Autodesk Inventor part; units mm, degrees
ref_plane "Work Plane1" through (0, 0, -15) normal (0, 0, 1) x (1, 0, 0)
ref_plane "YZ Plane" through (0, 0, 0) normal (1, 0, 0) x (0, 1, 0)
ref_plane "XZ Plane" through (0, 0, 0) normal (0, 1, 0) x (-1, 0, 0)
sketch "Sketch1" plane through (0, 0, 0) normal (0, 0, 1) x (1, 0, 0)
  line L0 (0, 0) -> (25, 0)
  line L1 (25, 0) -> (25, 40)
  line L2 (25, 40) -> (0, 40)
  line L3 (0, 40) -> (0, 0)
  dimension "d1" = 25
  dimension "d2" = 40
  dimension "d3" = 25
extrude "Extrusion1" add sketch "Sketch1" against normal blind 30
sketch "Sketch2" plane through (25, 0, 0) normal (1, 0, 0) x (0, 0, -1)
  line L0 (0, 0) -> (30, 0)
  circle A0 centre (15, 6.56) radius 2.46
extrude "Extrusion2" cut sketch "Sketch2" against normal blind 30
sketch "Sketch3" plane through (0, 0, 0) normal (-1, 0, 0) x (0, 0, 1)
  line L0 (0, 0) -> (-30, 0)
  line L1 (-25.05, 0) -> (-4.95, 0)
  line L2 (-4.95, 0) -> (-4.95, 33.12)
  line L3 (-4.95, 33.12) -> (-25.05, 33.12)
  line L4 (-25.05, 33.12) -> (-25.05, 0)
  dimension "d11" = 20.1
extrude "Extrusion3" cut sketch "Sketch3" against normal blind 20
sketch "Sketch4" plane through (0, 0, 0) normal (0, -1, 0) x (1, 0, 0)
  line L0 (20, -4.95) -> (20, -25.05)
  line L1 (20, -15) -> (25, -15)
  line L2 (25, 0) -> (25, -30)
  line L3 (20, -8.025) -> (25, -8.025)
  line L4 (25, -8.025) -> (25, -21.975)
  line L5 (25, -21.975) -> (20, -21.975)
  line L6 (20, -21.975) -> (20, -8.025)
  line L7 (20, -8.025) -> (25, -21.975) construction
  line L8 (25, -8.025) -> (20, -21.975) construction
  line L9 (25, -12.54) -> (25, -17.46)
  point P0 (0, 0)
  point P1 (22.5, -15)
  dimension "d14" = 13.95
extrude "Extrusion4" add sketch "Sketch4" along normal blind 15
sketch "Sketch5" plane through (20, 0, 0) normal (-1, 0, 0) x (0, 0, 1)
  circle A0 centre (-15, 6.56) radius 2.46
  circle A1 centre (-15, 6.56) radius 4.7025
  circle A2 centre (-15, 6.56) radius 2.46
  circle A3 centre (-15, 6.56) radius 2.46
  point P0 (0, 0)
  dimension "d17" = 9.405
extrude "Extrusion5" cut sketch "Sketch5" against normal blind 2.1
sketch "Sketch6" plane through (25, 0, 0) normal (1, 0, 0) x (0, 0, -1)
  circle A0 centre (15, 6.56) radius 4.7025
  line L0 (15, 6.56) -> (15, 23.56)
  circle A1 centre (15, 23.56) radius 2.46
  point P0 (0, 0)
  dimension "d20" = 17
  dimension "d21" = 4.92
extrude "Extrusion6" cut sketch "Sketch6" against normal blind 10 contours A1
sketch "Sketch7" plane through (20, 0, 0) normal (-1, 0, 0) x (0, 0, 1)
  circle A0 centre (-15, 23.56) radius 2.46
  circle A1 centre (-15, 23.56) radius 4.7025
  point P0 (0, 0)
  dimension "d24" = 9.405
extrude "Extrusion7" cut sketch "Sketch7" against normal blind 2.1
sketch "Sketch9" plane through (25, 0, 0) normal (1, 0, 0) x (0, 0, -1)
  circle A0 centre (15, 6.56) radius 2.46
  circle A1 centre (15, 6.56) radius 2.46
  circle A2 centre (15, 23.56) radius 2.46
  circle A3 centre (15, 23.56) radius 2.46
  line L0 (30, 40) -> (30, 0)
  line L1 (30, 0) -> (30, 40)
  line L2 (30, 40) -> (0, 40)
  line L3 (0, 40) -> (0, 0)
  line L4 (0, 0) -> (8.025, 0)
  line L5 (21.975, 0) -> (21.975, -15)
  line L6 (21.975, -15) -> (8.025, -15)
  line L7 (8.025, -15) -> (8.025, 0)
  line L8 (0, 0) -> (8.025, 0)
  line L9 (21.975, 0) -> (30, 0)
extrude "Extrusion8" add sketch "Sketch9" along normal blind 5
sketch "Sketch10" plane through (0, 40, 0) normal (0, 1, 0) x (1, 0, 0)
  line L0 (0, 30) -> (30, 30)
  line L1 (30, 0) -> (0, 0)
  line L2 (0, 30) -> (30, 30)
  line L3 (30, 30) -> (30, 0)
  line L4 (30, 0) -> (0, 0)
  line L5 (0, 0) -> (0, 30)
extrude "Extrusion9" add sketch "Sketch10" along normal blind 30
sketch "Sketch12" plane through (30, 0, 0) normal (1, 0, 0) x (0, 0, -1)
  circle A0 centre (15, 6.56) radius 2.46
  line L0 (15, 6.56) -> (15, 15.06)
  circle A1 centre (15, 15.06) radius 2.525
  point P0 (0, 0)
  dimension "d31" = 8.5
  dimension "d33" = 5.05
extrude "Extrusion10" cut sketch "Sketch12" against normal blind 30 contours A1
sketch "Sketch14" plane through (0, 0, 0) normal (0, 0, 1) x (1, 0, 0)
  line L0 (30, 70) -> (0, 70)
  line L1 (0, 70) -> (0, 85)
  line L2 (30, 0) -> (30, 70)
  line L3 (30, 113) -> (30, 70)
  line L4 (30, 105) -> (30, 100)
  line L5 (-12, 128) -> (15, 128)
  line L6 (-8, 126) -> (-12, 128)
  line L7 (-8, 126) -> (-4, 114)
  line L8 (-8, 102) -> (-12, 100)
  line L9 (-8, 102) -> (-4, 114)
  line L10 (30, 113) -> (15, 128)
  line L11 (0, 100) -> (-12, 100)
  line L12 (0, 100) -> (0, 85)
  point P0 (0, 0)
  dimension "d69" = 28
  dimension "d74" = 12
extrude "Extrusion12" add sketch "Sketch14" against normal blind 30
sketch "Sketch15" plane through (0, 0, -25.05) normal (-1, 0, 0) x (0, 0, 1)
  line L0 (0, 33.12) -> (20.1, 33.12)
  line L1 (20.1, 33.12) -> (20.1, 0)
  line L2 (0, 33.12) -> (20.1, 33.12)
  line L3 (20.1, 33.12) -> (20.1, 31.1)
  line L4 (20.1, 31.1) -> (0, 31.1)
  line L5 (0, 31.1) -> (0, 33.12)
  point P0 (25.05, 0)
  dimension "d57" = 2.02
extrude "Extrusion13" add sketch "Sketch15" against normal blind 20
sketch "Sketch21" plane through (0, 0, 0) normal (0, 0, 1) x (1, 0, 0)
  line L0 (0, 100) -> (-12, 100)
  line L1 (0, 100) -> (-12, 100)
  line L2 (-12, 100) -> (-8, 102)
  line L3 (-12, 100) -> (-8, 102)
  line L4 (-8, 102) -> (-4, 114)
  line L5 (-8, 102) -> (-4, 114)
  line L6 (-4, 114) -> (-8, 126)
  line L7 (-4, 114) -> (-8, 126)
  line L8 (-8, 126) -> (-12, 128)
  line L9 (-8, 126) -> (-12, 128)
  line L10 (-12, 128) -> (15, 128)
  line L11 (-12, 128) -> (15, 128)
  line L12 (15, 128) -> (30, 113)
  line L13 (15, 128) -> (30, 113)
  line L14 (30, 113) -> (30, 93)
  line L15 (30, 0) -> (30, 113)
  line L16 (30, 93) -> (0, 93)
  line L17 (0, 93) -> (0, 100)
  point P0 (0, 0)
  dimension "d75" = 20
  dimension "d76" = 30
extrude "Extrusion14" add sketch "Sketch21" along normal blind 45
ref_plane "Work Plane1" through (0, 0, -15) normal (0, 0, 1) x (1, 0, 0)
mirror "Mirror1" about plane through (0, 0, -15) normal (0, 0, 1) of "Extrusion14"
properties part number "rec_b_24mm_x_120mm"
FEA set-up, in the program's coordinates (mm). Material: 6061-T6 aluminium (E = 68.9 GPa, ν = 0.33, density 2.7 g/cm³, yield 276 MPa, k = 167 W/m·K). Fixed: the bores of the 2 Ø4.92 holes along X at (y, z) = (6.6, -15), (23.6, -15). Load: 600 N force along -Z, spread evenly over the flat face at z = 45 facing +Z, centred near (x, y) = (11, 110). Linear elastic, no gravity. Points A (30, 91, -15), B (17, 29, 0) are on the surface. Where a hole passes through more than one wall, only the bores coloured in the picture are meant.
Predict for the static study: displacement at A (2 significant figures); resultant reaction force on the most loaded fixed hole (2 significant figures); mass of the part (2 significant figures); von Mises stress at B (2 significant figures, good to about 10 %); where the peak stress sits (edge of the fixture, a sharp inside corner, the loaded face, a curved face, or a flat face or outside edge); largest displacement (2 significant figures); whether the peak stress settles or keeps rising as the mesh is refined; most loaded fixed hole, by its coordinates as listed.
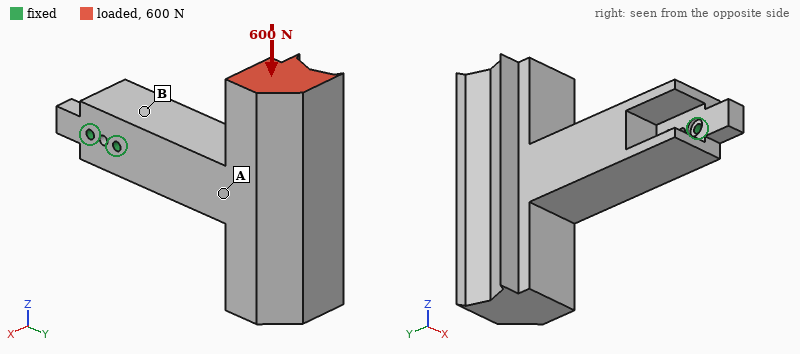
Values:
0.066 mm
2.8 kN
560 g
18 MPa
edge of the fixture
0.14 mm
keeps rising
(23.6, -15)
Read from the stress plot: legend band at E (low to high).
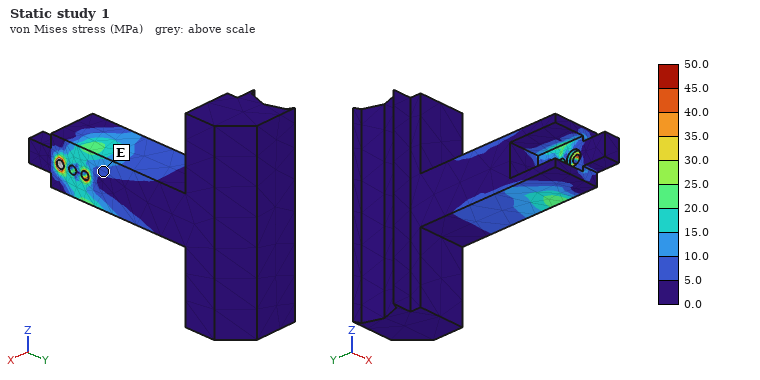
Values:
5.0 to 10.0 MPa
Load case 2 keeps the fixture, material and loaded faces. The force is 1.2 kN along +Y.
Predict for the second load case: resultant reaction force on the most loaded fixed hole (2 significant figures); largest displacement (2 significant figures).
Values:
3.3 kN
0.25 mm
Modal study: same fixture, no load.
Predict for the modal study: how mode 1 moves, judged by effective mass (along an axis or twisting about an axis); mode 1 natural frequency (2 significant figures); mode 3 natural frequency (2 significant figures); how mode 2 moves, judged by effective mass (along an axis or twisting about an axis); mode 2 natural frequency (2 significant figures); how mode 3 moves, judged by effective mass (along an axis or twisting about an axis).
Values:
along X
540 Hz
860 Hz
along Z
590 Hz
twisting about Y
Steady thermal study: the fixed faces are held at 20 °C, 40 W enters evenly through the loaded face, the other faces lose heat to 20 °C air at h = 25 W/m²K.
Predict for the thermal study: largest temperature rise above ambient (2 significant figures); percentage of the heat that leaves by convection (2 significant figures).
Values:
31 K
32 %
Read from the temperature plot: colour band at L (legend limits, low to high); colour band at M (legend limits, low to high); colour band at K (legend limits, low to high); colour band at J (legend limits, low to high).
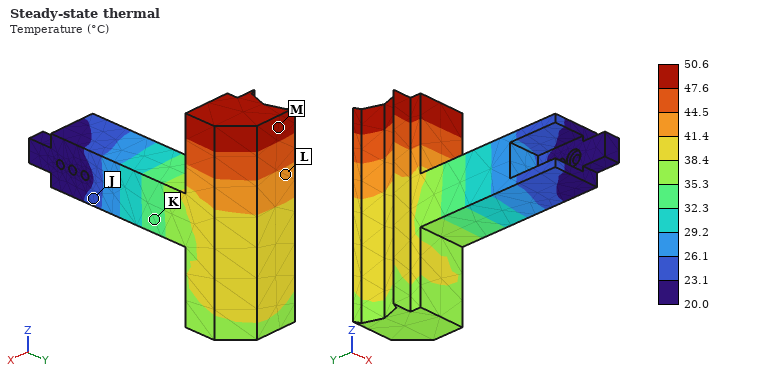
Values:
41.4 to 44.5 °C
47.6 to 50.6 °C
32.3 to 35.3 °C
23.1 to 26.1 °C
